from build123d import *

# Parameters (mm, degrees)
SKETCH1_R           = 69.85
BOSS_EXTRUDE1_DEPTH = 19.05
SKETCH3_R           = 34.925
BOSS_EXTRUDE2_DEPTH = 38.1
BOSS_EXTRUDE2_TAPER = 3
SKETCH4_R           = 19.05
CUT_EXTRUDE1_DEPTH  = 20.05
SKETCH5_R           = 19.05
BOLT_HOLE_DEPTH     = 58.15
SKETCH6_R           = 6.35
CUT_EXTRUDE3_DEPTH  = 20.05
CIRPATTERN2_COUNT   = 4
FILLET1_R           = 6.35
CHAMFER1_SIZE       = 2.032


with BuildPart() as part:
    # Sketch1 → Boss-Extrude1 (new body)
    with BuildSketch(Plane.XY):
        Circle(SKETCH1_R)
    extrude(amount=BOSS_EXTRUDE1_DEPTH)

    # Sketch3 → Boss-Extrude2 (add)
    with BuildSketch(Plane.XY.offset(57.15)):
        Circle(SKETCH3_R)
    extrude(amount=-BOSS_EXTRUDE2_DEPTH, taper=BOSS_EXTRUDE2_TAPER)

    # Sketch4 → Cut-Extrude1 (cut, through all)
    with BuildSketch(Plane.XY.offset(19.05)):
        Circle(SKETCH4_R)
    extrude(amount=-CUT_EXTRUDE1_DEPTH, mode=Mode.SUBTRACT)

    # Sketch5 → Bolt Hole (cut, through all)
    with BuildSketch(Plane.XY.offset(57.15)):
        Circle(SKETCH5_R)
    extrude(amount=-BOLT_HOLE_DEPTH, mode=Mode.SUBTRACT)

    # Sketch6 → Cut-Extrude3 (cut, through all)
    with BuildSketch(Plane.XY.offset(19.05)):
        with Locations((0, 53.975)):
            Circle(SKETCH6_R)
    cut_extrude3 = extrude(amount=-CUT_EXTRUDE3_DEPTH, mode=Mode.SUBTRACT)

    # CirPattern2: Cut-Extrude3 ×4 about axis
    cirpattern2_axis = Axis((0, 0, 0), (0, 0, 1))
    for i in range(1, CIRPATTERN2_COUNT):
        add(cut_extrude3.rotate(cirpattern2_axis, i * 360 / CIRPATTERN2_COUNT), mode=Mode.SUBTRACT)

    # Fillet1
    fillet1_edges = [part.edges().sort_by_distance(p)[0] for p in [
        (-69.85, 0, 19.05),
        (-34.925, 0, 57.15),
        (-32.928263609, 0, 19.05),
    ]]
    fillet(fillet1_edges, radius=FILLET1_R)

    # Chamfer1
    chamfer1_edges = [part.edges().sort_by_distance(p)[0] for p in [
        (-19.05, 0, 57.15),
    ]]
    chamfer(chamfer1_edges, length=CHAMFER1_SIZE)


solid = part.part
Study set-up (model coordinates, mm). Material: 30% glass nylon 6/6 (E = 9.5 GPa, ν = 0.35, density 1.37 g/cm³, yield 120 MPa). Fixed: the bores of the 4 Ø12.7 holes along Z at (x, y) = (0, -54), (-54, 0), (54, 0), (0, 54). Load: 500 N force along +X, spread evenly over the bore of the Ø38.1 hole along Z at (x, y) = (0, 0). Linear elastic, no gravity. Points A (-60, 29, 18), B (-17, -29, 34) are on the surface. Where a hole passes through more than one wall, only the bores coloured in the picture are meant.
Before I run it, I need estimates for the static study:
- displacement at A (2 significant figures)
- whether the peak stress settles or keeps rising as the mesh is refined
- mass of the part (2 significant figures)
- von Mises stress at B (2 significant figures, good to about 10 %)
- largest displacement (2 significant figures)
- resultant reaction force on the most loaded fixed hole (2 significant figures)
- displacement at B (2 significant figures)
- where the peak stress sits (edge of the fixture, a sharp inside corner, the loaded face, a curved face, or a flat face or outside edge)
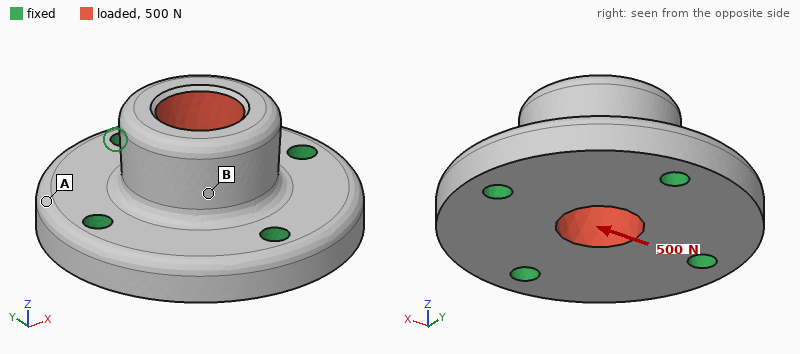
0.53 µm
keeps rising
480 g
0.15 MPa
3.4 µm
180 N
1.9 µm
edge of the fixture
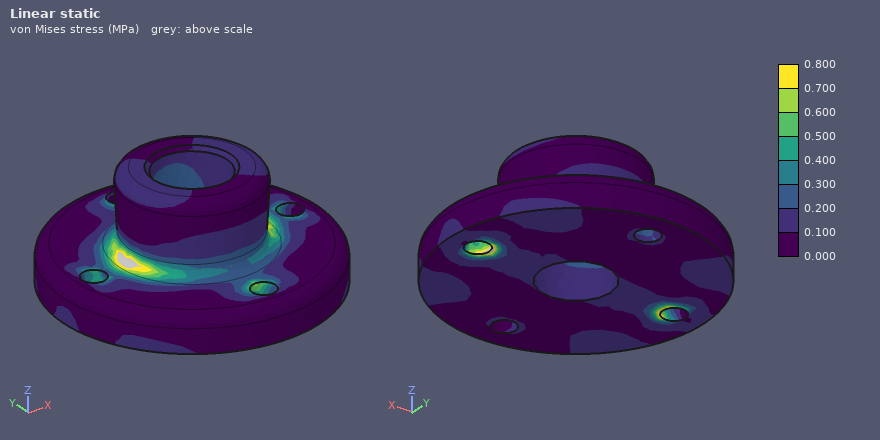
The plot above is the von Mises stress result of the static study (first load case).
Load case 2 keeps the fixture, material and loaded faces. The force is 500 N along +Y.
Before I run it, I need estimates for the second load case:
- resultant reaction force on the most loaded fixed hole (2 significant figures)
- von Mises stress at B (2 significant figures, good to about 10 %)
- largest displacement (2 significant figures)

180 N
0.10 MPa
3.4 µm
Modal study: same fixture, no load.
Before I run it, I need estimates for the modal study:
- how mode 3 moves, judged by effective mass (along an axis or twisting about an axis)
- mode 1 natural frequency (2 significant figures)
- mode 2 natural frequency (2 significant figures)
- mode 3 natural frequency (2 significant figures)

along Z
4600 Hz
4600 Hz
5000 Hz
